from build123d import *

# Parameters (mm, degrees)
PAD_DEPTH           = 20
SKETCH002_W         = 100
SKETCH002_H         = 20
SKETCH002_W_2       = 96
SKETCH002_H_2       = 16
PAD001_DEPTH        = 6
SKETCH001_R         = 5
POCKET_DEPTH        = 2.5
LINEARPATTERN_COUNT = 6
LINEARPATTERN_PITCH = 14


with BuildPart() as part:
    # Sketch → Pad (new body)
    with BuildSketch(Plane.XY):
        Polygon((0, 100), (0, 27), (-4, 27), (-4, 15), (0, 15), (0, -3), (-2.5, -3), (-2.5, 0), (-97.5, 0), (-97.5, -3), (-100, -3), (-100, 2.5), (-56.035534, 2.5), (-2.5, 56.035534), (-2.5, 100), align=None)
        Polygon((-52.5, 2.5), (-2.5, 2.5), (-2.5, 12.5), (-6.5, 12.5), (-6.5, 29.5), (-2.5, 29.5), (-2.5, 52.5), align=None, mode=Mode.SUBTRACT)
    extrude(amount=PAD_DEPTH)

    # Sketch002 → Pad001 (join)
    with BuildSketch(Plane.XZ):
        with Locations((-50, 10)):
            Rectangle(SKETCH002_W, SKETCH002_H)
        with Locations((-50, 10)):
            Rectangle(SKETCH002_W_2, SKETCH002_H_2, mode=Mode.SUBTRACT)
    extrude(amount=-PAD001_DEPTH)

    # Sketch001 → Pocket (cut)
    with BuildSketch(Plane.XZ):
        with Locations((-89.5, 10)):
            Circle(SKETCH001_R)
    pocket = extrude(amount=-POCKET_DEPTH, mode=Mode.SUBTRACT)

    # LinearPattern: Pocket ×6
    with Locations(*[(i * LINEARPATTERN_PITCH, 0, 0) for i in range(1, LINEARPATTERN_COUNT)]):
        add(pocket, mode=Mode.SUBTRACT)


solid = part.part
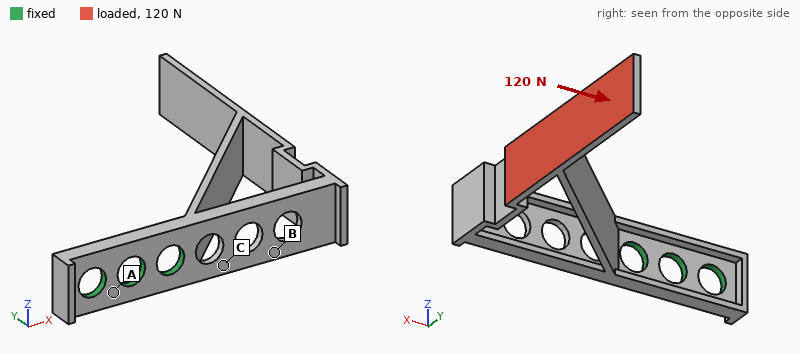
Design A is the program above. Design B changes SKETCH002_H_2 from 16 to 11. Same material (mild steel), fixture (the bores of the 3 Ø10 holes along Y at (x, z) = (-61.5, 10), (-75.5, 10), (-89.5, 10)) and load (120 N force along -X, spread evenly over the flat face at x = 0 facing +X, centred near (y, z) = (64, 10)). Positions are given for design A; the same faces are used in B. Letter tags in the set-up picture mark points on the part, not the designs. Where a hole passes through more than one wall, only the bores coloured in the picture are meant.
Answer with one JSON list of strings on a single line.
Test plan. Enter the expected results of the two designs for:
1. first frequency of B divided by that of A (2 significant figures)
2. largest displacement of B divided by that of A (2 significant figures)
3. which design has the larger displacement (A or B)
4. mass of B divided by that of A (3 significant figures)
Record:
["1.2", "0.75", "A", "1.11"]
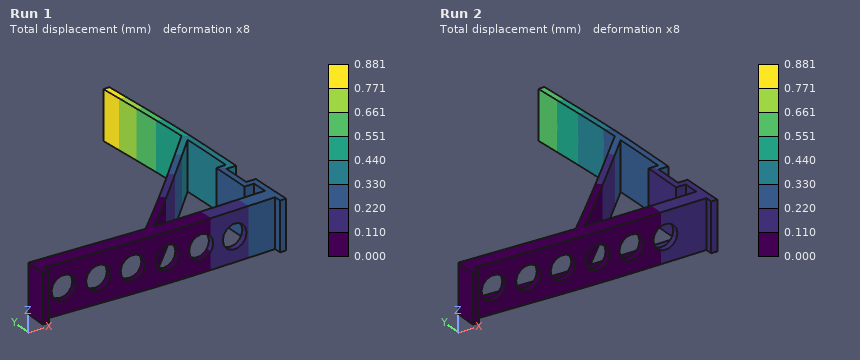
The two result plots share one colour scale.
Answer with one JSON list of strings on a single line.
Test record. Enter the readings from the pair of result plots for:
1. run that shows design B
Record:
["Run 2"]
